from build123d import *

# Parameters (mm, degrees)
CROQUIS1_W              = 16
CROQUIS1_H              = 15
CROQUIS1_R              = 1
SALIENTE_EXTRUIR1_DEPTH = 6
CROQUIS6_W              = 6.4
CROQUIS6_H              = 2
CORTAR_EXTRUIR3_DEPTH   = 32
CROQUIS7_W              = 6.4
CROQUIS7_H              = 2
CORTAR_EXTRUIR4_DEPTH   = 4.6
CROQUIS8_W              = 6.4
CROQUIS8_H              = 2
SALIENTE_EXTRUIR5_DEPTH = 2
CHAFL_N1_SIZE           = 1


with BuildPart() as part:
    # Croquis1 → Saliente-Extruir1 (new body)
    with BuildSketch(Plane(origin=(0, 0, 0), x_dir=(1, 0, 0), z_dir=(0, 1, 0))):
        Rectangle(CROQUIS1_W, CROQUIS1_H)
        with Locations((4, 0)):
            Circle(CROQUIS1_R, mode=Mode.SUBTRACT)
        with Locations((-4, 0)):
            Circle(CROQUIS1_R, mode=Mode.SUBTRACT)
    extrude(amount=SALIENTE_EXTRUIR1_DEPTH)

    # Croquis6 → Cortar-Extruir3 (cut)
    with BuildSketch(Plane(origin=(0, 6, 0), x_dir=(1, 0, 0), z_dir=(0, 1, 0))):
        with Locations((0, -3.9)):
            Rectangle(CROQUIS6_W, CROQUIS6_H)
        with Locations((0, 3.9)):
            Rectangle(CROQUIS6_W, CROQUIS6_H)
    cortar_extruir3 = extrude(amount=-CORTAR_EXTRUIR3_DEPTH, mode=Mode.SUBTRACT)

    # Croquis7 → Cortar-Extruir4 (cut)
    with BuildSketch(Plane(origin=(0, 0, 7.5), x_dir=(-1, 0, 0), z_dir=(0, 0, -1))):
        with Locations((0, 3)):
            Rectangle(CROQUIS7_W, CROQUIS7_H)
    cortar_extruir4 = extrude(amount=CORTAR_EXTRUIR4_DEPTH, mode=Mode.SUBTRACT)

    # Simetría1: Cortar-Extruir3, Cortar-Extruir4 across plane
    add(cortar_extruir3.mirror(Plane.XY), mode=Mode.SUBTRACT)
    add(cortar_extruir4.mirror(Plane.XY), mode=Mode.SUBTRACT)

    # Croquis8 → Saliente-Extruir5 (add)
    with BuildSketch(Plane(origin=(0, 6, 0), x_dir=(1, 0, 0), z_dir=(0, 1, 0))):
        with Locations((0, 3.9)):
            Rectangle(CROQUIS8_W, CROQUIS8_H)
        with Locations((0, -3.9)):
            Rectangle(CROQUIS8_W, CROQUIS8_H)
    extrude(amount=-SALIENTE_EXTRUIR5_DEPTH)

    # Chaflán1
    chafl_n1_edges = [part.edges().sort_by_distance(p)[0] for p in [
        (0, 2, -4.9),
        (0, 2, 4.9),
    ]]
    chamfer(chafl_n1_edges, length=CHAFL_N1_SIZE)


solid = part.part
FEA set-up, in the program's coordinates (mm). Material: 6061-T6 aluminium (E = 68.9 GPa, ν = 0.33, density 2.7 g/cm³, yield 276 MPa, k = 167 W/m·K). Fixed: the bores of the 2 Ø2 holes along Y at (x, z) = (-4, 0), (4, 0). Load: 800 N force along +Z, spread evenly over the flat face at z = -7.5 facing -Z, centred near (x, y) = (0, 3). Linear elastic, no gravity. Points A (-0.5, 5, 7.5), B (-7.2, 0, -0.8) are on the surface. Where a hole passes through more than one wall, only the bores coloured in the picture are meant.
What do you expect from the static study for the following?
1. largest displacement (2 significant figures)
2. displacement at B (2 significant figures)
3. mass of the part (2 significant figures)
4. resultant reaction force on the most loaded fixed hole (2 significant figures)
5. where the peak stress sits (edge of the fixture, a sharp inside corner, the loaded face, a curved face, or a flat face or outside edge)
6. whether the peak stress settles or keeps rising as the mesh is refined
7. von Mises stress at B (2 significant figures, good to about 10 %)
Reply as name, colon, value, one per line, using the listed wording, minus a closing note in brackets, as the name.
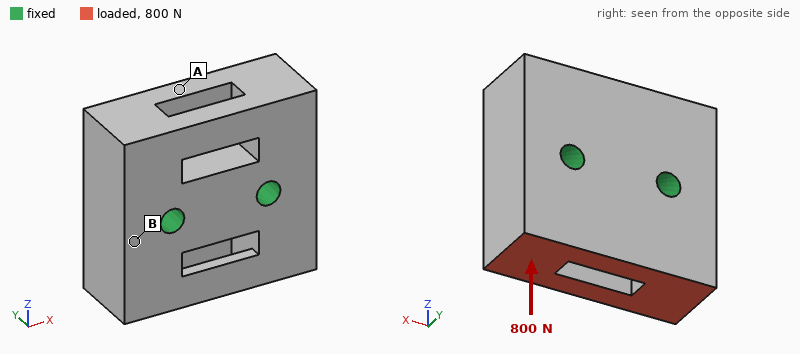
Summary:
largest displacement: 4.2 µm
displacement at B: 0.67 µm
mass of the part: 3.3 g
resultant reaction force on the most loaded fixed hole: 400 N
where the peak stress sits: a sharp inside corner
whether the peak stress settles or keeps rising as the mesh is refined: keeps rising
von Mises stress at B: 7.6 MPa
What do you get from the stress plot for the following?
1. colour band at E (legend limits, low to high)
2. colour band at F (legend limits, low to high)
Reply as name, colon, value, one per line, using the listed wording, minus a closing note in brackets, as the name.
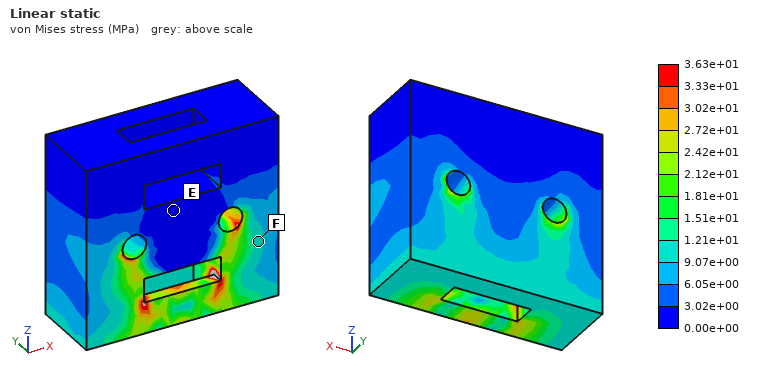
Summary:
colour band at E: 0.00e+00 to 3.02e+00 MPa
colour band at F: 9.07e+00 to 1.21e+01 MPa
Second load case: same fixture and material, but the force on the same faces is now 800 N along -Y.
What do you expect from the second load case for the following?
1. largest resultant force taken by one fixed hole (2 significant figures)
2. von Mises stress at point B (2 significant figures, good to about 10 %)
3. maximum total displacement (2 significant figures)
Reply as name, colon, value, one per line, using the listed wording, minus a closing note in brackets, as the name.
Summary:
largest resultant force taken by one fixed hole: 400 N
von Mises stress at point B: 39 MPa
maximum total displacement: 19 µm
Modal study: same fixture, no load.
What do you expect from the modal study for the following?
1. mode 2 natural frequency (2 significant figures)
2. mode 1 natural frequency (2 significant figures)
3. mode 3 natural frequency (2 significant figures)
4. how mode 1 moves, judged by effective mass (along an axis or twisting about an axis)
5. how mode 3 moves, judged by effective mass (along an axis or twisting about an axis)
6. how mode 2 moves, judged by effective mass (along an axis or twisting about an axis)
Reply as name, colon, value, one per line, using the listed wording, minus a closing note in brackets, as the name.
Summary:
mode 2 natural frequency: 56 kHz
mode 1 natural frequency: 53 kHz
mode 3 natural frequency: 62 kHz
how mode 1 moves, judged by effective mass: twisting about X
how mode 3 moves, judged by effective mass: along Y
how mode 2 moves, judged by effective mass: twisting about Y
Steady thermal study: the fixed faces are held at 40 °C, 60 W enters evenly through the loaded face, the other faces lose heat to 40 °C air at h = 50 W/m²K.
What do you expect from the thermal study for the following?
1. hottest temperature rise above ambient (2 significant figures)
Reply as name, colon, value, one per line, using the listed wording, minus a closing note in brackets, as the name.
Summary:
hottest temperature rise above ambient: 49 K
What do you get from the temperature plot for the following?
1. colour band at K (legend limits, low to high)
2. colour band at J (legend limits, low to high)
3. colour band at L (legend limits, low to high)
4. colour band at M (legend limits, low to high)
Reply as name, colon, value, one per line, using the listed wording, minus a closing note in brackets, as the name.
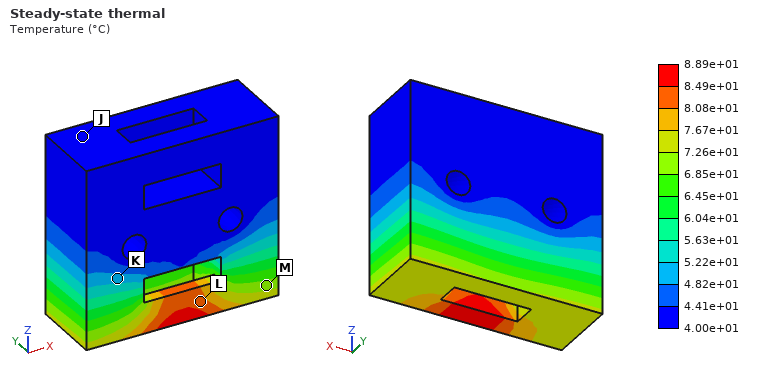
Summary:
colour band at K: 4.82e+01 to 5.22e+01 °C
colour band at J: 4.00e+01 to 4.41e+01 °C
colour band at L: 8.08e+01 to 8.49e+01 °C
colour band at M: 6.85e+01 to 7.26e+01 °C
